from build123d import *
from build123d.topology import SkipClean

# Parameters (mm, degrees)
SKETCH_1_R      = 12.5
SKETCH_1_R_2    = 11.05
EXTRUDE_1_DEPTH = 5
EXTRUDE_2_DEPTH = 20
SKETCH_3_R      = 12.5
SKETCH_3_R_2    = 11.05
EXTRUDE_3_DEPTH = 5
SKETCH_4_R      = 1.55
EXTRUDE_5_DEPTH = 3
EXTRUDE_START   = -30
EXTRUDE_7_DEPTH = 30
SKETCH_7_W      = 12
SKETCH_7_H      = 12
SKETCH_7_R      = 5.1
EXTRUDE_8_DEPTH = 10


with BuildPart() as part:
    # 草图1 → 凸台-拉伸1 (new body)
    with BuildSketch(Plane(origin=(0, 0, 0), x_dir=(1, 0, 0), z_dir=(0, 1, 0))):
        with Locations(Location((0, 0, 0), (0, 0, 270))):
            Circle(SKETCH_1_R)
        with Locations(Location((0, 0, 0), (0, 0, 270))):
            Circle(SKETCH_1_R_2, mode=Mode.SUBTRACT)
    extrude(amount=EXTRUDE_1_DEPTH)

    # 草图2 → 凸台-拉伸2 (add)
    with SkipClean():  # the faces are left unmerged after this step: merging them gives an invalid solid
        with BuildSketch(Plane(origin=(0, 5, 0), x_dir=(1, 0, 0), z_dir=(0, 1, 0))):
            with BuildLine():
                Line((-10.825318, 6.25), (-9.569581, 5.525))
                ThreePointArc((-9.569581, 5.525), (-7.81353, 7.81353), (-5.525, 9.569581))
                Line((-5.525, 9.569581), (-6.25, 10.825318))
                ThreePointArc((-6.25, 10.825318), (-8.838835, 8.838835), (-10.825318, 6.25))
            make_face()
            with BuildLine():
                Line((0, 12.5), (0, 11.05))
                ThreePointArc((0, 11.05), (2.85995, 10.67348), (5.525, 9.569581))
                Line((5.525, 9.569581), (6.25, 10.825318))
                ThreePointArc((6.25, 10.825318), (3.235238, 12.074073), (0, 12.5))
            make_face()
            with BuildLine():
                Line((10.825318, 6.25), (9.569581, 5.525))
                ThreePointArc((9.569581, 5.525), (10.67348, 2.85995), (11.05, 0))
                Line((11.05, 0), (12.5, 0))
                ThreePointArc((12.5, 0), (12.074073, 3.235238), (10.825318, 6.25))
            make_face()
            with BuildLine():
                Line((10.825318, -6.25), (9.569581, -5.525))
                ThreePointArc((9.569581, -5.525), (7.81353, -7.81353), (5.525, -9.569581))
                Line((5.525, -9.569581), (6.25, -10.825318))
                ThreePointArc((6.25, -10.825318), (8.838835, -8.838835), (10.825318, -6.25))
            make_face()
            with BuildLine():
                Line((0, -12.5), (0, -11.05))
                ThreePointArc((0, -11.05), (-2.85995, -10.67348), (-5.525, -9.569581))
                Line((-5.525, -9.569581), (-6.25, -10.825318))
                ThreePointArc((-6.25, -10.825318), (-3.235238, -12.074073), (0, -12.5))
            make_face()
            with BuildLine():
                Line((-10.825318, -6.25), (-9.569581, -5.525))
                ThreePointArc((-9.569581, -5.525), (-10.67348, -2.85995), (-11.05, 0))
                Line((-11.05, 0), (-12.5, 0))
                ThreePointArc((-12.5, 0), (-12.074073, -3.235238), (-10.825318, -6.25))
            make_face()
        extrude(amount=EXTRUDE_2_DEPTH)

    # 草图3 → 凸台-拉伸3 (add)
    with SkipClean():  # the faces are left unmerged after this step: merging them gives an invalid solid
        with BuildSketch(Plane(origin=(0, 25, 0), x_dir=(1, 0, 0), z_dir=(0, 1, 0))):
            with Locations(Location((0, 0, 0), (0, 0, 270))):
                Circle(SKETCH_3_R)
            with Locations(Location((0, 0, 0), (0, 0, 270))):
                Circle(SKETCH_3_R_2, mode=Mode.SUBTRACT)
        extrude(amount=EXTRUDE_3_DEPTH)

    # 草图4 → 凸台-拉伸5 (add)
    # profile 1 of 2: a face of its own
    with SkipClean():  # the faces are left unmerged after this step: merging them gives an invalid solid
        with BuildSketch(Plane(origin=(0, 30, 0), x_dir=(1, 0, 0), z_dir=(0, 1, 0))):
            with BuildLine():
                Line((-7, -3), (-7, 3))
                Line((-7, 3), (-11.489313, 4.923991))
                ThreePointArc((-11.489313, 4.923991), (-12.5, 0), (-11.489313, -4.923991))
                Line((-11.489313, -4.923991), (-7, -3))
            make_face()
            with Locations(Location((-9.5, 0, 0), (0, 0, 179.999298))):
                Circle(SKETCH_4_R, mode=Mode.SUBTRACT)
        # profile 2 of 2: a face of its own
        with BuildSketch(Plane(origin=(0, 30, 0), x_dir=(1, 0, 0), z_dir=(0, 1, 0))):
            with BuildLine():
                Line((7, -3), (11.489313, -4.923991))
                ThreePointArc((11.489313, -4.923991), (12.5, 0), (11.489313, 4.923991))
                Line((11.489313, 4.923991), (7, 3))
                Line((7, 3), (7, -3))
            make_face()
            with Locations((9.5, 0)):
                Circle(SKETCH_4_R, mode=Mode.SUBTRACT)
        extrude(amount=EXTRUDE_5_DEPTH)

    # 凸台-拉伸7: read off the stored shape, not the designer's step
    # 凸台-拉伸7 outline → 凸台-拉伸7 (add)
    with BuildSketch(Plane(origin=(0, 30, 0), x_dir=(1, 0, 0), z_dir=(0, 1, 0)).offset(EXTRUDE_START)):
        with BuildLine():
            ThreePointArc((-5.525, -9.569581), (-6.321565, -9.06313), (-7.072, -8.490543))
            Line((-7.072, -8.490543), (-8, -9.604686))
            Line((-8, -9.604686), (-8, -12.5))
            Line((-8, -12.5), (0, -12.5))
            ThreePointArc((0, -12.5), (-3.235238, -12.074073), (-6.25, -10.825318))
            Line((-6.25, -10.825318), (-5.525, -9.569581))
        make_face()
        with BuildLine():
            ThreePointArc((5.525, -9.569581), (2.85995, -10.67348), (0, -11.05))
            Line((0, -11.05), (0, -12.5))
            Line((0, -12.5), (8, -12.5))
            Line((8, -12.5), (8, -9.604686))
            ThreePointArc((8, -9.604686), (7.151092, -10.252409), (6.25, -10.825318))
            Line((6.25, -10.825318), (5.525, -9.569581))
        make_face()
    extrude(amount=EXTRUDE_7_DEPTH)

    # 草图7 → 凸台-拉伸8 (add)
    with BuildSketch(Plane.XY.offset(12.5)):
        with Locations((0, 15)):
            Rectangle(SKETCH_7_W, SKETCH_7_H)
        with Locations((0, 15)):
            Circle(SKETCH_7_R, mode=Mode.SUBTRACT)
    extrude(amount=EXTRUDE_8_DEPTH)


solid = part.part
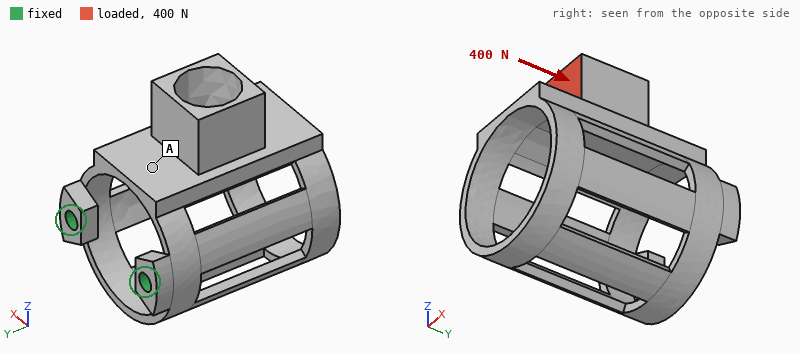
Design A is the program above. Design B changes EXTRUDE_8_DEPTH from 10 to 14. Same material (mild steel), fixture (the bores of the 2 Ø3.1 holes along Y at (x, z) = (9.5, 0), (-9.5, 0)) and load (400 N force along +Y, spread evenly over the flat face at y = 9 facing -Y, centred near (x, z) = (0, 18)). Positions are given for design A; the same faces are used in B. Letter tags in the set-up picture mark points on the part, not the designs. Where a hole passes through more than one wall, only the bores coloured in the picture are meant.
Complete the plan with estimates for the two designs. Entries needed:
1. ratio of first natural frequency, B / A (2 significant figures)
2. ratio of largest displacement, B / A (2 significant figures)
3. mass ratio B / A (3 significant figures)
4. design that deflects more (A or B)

0.93
1.2
1.07
B
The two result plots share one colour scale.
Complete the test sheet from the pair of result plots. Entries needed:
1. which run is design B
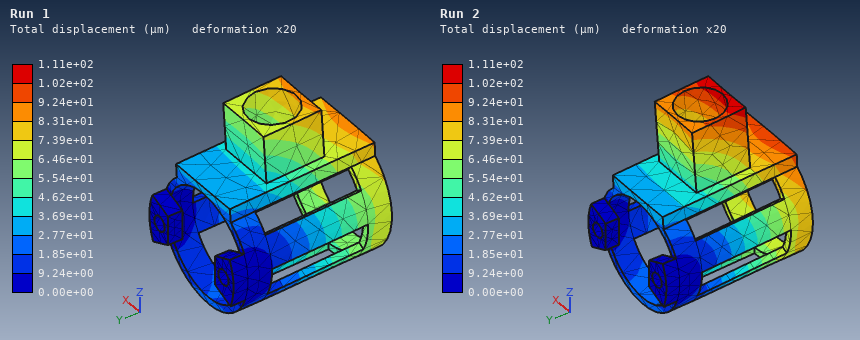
Run 2
